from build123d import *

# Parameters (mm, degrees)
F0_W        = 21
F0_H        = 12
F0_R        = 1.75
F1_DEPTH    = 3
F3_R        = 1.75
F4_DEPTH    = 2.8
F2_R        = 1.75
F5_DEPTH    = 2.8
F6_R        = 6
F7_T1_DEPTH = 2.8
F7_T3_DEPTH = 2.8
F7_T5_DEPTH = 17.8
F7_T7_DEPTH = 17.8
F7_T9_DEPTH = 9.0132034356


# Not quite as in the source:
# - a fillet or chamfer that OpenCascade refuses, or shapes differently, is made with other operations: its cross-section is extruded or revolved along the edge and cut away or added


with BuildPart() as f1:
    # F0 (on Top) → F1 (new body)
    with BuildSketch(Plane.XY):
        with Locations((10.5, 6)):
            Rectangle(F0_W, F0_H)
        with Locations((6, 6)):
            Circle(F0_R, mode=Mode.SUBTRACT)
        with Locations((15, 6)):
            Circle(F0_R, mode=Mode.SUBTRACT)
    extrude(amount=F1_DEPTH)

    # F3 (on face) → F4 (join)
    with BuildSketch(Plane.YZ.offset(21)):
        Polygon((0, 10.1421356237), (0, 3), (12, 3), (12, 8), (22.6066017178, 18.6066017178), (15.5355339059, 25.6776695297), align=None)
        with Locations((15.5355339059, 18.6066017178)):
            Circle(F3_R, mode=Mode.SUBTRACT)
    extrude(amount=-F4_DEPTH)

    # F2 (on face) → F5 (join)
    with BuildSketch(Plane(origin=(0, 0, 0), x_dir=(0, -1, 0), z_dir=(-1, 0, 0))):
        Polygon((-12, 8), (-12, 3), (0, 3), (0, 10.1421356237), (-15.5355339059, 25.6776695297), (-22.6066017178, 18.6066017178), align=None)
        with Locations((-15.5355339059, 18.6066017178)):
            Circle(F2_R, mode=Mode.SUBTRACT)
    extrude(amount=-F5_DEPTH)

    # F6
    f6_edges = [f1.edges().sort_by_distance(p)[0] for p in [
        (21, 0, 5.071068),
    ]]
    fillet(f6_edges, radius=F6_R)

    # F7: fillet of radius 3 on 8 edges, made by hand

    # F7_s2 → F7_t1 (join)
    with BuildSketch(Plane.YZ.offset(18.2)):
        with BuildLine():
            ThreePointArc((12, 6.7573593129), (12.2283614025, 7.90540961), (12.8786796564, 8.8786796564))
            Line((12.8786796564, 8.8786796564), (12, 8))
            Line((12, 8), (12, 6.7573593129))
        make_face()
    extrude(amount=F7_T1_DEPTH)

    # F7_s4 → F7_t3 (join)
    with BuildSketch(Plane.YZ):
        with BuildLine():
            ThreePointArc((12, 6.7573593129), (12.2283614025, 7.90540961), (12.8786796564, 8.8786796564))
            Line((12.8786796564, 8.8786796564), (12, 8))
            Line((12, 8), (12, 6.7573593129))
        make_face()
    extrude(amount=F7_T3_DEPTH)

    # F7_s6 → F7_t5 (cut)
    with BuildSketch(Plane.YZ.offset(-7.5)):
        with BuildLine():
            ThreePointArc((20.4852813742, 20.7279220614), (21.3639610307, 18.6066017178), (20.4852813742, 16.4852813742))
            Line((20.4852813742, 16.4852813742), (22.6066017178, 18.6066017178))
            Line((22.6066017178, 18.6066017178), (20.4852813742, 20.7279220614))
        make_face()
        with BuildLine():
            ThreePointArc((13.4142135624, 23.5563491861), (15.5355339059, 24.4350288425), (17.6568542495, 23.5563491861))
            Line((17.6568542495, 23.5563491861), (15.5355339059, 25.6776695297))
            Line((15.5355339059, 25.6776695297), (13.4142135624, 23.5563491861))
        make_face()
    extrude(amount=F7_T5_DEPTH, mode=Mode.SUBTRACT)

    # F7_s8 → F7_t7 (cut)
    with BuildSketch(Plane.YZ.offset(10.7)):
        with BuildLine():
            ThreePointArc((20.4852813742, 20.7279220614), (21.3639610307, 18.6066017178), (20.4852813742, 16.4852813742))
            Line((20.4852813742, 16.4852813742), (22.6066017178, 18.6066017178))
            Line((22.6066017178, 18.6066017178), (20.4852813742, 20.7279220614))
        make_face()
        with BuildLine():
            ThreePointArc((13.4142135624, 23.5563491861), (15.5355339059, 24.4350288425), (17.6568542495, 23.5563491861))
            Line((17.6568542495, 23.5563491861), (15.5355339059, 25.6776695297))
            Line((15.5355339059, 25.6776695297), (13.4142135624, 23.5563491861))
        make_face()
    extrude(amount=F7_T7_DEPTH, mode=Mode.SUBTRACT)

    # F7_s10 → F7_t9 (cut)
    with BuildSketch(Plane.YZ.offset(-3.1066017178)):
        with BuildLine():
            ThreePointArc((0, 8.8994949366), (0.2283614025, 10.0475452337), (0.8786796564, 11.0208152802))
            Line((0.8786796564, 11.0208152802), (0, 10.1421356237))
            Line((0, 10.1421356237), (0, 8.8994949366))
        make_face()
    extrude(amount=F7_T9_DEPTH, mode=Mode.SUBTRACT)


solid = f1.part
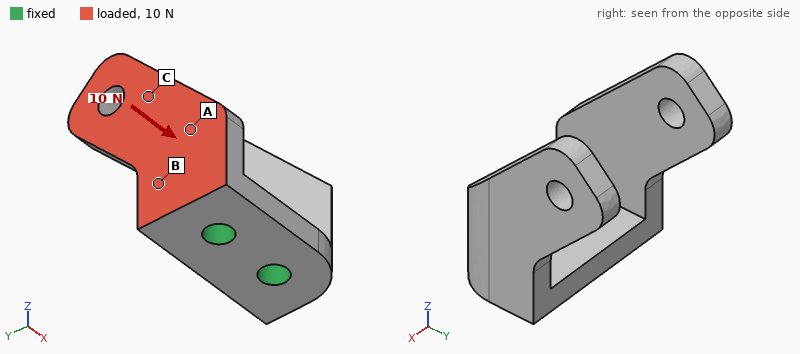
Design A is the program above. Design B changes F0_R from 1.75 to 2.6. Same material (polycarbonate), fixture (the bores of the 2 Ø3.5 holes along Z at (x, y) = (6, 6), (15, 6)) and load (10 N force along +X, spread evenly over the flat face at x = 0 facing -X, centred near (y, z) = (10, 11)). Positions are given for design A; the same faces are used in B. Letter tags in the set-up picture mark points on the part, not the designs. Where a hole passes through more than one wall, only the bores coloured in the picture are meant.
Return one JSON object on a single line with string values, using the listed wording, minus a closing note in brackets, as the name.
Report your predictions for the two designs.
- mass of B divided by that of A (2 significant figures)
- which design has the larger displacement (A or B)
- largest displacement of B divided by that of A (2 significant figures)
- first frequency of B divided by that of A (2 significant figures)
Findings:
{"mass of B divided by that of A": "0.96", "which design has the larger displacement": "A", "largest displacement of B divided by that of A": "0.91", "first frequency of B divided by that of A": "1.0"}
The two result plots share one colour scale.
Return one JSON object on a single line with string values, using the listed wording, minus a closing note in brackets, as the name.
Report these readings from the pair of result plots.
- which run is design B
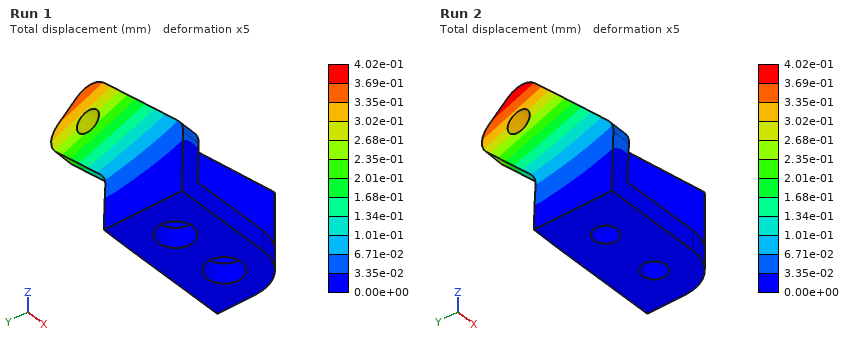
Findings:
{"which run is design B": "Run 1"}
